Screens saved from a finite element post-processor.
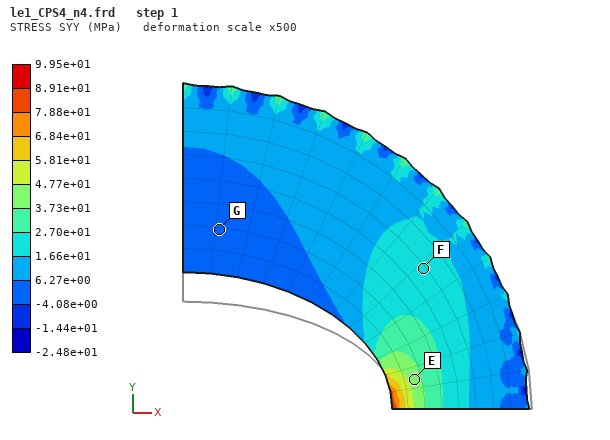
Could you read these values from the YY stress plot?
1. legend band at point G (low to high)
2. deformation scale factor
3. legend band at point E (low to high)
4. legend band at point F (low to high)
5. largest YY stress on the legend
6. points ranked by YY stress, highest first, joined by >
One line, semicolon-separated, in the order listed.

-4.08e+00 to 6.27e+00 MPa; 500; 3.73e+01 to 4.77e+01 MPa; 1.66e+01 to 2.70e+01 MPa; 9.95e+01 MPa; E > F > G
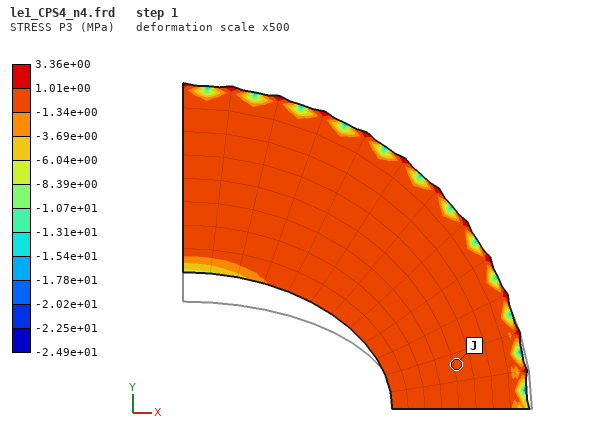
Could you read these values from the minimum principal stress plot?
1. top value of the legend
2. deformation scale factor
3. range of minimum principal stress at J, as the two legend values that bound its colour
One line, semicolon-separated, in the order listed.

3.36e+00 MPa; 500; -1.34e+00 to 1.01e+00 MPa
